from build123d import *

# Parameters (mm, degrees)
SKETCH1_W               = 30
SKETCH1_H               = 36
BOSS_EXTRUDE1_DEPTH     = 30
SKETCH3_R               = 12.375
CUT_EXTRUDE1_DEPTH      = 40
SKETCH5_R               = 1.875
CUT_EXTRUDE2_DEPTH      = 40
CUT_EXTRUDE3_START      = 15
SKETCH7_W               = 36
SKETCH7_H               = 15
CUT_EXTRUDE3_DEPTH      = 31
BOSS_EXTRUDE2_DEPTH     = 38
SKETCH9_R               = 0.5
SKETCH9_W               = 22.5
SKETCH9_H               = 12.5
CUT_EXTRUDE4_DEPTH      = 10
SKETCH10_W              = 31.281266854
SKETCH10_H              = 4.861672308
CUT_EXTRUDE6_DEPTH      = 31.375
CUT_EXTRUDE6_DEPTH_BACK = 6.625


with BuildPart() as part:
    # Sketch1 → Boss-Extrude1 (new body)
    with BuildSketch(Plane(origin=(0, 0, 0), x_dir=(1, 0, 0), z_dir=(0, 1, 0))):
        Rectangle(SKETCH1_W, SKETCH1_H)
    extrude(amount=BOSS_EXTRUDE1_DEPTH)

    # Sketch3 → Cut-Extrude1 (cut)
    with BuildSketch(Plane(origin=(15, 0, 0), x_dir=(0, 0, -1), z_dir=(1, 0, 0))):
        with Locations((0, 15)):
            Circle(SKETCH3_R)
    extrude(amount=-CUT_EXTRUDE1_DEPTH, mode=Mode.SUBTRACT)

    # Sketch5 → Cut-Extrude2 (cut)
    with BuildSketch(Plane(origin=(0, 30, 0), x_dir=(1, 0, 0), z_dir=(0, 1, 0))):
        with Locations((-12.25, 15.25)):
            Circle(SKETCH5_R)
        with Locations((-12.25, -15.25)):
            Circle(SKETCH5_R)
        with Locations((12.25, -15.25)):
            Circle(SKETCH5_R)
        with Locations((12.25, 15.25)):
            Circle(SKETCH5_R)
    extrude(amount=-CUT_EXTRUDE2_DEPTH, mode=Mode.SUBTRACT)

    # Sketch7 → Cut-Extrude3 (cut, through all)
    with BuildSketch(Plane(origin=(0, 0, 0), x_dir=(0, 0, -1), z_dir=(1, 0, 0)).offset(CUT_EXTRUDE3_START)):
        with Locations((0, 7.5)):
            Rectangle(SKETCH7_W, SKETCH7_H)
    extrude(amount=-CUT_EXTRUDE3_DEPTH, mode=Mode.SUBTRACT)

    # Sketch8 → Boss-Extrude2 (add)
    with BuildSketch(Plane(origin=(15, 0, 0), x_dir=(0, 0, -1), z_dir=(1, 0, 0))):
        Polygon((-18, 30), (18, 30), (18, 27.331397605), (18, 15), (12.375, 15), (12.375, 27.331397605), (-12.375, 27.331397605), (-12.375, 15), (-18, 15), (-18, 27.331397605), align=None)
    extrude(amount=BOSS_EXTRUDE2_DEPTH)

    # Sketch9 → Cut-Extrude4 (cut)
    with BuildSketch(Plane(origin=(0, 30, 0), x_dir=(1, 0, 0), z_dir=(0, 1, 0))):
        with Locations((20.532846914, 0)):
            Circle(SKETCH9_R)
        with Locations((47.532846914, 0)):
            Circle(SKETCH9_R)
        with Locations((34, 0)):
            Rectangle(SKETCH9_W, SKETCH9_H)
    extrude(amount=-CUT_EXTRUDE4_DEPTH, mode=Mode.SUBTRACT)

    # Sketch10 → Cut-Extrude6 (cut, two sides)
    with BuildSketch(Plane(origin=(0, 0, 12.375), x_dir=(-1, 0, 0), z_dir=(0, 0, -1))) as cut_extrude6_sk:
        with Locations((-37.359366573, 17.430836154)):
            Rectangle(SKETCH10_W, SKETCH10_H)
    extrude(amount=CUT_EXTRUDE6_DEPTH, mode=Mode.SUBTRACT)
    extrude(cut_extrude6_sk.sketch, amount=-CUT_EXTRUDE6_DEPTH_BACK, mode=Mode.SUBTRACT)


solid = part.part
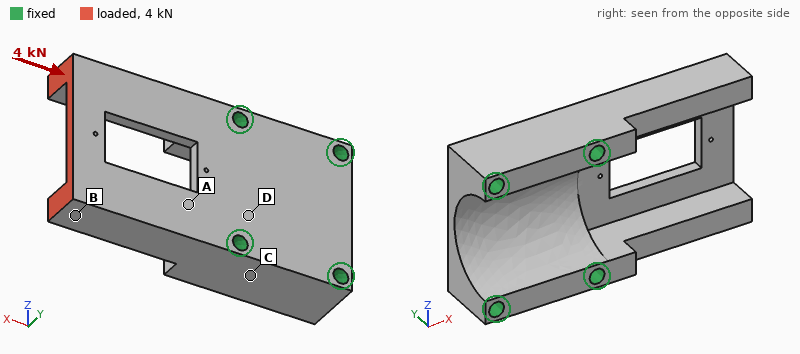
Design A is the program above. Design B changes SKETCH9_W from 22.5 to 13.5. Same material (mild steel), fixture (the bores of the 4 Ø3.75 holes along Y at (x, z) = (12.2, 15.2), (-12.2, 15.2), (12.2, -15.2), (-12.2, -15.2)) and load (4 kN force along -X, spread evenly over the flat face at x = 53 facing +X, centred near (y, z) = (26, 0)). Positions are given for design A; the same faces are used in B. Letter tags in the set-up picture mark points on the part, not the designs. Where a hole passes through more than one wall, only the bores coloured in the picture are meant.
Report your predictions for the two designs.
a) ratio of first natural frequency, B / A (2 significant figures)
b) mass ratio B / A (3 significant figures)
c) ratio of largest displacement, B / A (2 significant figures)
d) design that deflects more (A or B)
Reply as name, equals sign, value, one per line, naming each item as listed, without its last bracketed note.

ratio of first natural frequency, B / A = 0.98
mass ratio B / A = 1.02
ratio of largest displacement, B / A = 0.85
design that deflects more = A
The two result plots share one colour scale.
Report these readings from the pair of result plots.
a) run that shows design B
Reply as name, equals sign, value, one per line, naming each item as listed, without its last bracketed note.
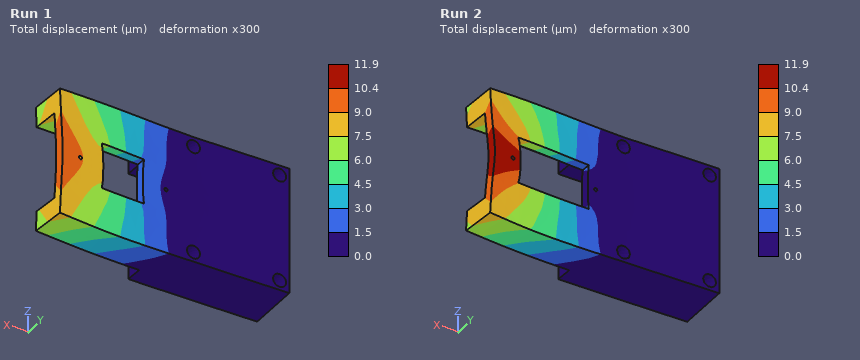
run that shows design B = Run 1
